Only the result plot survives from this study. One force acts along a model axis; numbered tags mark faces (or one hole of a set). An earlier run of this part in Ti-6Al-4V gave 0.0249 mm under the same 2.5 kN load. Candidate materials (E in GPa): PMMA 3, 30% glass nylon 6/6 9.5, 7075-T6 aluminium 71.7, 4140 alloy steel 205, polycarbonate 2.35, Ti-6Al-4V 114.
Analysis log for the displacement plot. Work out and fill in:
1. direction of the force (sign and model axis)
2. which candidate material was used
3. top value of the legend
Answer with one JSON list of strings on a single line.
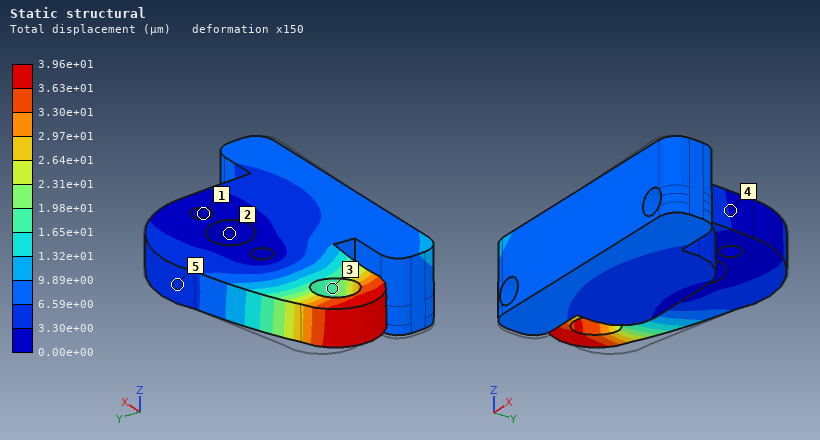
["-Y", "7075-T6 aluminium", "3.96e+01 µm"]
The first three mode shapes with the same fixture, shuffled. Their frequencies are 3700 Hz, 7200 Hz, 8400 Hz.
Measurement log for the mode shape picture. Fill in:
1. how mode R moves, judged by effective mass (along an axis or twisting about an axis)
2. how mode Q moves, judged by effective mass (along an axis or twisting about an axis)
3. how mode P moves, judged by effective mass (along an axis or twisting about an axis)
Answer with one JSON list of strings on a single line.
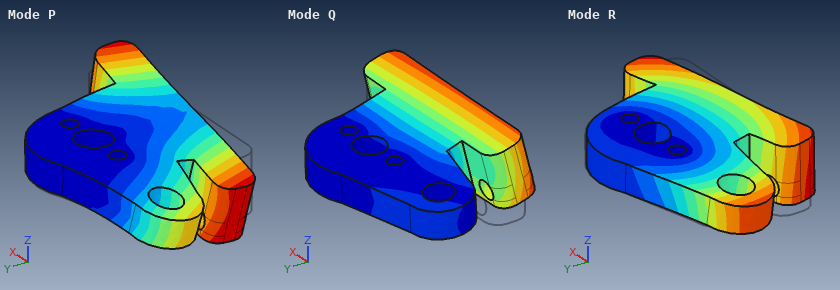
["along X", "along Z", "twisting about Y"]
